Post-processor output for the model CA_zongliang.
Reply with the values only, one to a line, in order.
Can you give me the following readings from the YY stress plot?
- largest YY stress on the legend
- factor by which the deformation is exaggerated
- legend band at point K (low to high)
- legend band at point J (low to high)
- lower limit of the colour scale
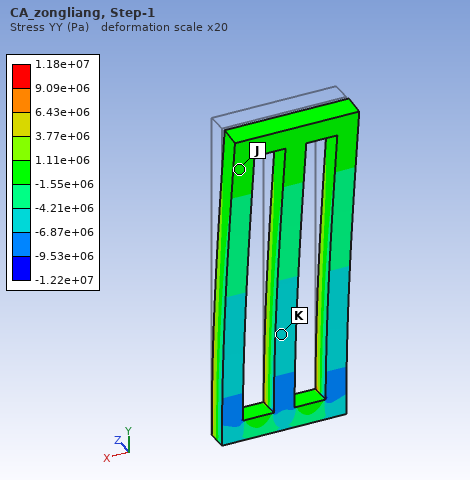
1.18e+07 Pa
20
-6.87e+06 to -4.21e+06 Pa
-1.55e+06 to 1.11e+06 Pa
-1.22e+07 Pa
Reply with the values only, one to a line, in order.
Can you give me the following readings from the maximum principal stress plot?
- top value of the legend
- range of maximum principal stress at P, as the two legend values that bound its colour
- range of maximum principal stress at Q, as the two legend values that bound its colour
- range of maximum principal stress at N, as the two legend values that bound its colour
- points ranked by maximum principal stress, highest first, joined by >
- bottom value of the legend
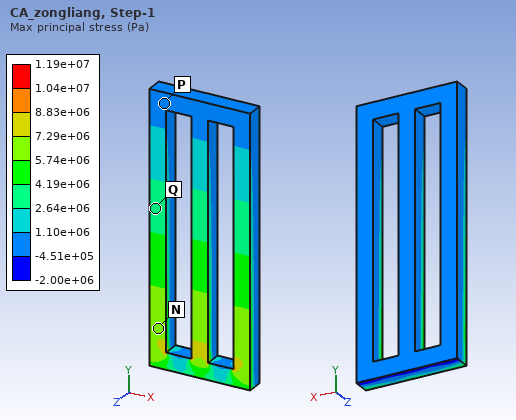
1.19e+07 Pa
-4.51e+05 to 1.10e+06 Pa
2.64e+06 to 4.19e+06 Pa
5.74e+06 to 7.29e+06 Pa
N > Q > P
-2.00e+06 Pa
